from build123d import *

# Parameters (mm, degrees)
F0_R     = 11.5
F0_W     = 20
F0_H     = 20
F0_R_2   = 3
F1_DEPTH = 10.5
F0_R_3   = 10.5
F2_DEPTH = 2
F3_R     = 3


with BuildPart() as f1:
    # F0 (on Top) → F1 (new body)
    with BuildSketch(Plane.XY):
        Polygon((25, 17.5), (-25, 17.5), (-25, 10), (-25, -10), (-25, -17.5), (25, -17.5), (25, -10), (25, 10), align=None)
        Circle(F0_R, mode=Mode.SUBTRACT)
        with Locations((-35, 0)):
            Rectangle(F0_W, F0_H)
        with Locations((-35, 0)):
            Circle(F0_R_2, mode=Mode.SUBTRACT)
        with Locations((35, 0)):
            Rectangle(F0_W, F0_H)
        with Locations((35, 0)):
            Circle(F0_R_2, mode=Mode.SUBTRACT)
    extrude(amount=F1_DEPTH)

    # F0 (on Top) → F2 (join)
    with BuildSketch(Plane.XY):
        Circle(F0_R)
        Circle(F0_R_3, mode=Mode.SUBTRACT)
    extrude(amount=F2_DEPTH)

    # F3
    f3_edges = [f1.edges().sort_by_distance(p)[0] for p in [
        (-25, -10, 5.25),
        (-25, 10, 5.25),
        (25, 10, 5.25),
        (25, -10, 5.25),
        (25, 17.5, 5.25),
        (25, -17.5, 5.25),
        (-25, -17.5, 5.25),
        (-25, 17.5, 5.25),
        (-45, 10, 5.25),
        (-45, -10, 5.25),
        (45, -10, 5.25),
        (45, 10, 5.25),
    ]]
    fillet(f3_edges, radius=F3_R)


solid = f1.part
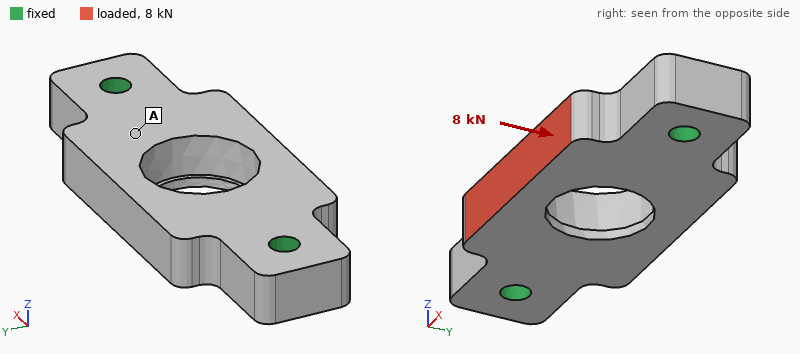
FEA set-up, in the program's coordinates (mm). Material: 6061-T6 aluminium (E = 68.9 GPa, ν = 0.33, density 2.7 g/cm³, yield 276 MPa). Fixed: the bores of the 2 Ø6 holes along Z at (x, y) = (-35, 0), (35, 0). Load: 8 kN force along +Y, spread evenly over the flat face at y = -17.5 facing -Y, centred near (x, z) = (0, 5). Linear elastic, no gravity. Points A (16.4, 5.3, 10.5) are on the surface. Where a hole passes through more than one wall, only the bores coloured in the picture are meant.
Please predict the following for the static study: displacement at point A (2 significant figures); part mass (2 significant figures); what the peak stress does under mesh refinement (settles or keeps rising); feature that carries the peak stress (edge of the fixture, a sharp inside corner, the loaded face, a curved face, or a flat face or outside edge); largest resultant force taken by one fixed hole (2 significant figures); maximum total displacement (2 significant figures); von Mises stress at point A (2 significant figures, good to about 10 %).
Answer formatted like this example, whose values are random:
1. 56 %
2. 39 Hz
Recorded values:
1. 19 µm
2. 59 g
3. keeps rising
4. edge of the fixture
5. 4.2 kN
6. 40 µm
7. 18 MPa
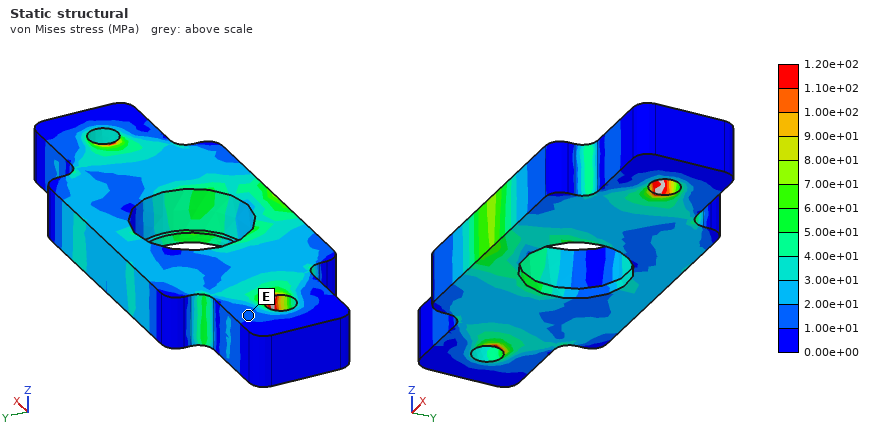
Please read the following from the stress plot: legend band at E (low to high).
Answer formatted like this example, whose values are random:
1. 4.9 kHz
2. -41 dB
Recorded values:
1. 1.00e+01 to 2.00e+01 MPa
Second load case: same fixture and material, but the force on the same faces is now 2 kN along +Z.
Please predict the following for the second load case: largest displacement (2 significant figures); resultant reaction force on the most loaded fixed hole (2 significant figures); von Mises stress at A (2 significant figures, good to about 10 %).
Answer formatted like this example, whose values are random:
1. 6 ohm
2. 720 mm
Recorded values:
1. 74 µm
2. 1.0 kN
3. 20 MPa
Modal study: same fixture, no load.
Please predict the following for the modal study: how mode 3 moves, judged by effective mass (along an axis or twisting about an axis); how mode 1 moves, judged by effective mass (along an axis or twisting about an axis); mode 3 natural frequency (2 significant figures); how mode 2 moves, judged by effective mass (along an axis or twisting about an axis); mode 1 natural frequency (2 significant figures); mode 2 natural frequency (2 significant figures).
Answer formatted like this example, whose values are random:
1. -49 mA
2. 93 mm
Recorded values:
1. along Y
2. along Z
3. 16 kHz
4. twisting about X
5. 9000 Hz
6. 9700 Hz
